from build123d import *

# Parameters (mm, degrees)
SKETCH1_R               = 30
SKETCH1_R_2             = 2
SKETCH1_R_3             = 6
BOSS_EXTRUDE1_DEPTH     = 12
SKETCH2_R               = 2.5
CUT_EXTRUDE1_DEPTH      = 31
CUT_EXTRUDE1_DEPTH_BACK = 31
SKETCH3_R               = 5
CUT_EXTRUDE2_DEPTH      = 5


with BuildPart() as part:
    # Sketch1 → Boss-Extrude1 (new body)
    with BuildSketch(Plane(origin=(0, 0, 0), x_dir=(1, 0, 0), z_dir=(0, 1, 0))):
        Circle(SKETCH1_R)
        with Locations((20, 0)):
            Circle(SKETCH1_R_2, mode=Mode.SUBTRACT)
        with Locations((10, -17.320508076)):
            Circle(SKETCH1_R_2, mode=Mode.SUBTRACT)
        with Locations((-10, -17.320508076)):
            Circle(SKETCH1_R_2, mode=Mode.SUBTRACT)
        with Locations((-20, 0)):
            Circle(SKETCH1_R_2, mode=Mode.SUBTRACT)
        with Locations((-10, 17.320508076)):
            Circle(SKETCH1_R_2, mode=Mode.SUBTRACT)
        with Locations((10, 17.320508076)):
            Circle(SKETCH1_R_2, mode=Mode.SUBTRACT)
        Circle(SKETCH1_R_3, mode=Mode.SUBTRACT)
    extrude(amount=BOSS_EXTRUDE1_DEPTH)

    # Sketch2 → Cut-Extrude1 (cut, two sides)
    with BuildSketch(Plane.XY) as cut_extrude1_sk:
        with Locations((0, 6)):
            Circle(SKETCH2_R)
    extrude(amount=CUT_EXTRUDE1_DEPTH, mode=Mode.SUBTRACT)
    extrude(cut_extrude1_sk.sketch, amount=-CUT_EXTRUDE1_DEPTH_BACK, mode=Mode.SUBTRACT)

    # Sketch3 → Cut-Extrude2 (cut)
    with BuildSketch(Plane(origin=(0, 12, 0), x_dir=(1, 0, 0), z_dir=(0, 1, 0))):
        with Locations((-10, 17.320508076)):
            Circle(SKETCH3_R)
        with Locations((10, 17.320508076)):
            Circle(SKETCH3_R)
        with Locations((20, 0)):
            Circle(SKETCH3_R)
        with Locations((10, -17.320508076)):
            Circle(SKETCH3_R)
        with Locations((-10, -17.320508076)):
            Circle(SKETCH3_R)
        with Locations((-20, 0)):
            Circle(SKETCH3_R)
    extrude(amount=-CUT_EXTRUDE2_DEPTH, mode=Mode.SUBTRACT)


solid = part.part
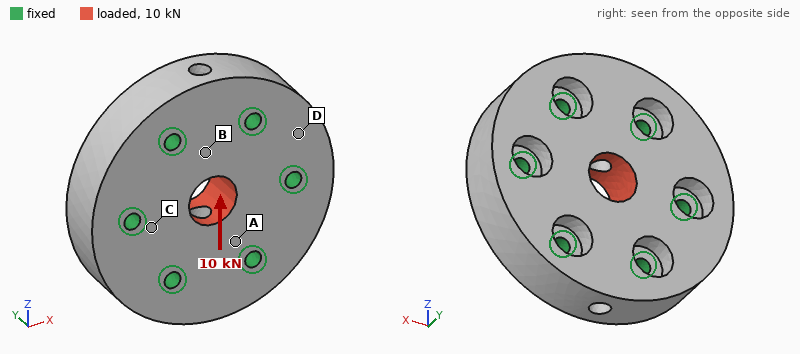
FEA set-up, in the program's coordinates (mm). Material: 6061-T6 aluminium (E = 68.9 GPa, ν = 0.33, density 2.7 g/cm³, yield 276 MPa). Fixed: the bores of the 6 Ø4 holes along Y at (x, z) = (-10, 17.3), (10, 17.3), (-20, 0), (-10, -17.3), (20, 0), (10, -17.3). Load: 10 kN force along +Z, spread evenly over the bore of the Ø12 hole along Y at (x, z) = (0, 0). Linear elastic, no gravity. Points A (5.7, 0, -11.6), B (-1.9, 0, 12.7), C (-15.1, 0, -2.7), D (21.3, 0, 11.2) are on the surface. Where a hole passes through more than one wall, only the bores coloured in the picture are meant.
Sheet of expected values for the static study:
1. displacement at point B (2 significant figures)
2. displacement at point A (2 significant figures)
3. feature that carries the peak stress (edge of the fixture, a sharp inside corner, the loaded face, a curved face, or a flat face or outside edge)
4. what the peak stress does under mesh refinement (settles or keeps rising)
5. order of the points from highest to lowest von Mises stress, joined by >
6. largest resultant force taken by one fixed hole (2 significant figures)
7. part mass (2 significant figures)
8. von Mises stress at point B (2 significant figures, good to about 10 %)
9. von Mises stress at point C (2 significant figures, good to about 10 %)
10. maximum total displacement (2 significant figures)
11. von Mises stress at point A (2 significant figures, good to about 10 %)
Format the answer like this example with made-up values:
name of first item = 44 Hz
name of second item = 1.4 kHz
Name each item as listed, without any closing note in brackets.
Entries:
displacement at point B = 2.8 µm
displacement at point A = 2.3 µm
feature that carries the peak stress = edge of the fixture
what the peak stress does under mesh refinement = keeps rising
order of the points from highest to lowest von Mises stress, joined by > = A > B > C > D
largest resultant force taken by one fixed hole = 2.1 kN
part mass = 78 g
von Mises stress at point B = 15 MPa
von Mises stress at point C = 7.8 MPa
maximum total displacement = 6.6 µm
von Mises stress at point A = 23 MPa
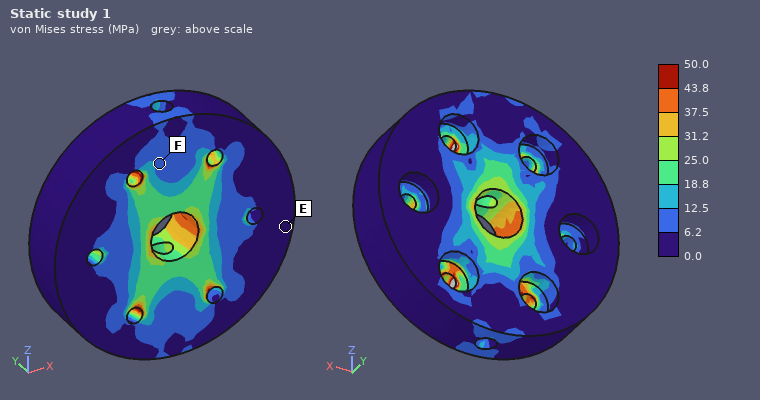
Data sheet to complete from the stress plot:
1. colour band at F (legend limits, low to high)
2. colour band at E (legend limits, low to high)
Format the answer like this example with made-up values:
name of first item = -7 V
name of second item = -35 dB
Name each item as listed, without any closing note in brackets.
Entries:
colour band at F = 6.2 to 12.5 MPa
colour band at E = 0.0 to 6.2 MPa
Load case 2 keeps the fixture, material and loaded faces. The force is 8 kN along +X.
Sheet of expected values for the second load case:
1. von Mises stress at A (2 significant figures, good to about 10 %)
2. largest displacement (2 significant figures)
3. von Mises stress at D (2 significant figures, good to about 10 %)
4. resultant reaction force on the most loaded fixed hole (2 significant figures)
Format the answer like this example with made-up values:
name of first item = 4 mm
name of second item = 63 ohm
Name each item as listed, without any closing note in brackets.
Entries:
von Mises stress at A = 12 MPa
largest displacement = 5.8 µm
von Mises stress at D = 5.0 MPa
resultant reaction force on the most loaded fixed hole = 2.0 kN
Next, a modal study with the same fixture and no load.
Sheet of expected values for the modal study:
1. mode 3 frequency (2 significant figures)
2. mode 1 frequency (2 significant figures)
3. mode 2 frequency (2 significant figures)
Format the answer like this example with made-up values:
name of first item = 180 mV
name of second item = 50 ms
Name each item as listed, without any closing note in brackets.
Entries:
mode 3 frequency = 30 kHz
mode 1 frequency = 29 kHz
mode 2 frequency = 30 kHz
